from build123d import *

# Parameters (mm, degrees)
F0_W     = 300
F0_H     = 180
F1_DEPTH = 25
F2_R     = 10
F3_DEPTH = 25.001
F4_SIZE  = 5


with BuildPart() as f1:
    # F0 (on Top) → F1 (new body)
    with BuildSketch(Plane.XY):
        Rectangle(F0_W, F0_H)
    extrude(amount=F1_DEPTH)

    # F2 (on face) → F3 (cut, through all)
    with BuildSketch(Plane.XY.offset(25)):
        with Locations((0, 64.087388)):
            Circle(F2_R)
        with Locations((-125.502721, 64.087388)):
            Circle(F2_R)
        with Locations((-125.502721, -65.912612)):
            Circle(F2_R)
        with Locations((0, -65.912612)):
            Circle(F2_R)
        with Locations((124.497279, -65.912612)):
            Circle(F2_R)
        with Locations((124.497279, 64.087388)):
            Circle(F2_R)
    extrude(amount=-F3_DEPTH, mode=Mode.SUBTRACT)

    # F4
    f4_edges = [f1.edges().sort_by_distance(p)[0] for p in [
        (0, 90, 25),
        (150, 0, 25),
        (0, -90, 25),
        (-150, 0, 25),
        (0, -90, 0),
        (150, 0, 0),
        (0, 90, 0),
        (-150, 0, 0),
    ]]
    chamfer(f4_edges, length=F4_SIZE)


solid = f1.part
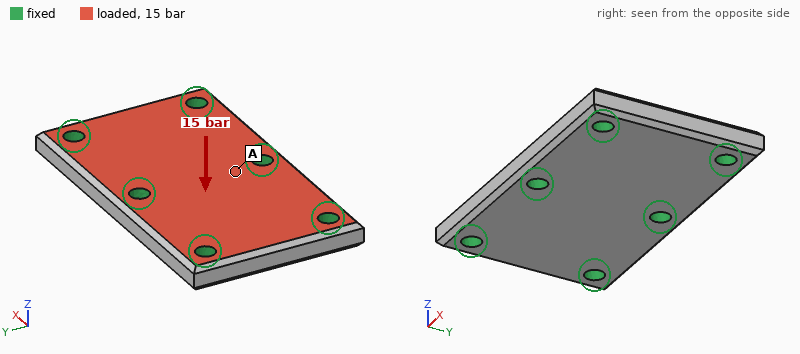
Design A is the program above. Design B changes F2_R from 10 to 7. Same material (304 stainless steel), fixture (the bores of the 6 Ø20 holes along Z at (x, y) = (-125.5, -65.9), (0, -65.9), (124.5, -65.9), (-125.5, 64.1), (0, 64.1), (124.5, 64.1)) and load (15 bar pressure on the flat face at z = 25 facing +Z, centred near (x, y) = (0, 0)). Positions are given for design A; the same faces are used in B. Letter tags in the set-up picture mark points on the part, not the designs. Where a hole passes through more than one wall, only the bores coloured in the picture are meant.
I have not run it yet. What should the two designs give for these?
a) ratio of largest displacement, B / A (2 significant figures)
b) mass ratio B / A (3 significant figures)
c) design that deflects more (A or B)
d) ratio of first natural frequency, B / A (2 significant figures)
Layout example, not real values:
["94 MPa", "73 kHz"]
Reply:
["1.2", "1.02", "B", "0.90"]
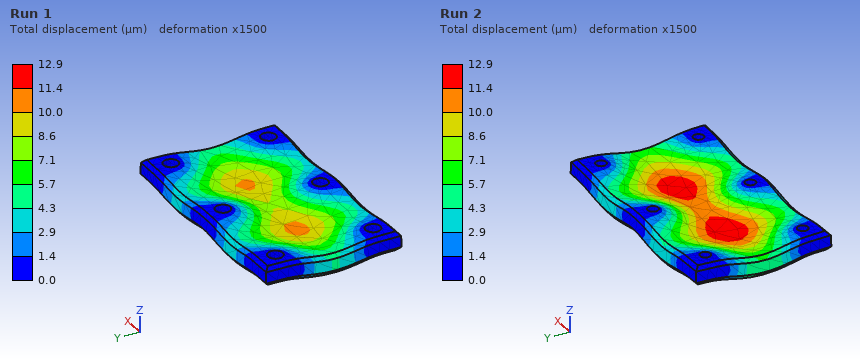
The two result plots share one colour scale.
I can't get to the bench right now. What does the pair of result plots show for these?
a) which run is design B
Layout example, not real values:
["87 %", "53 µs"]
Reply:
["Run 2"]
